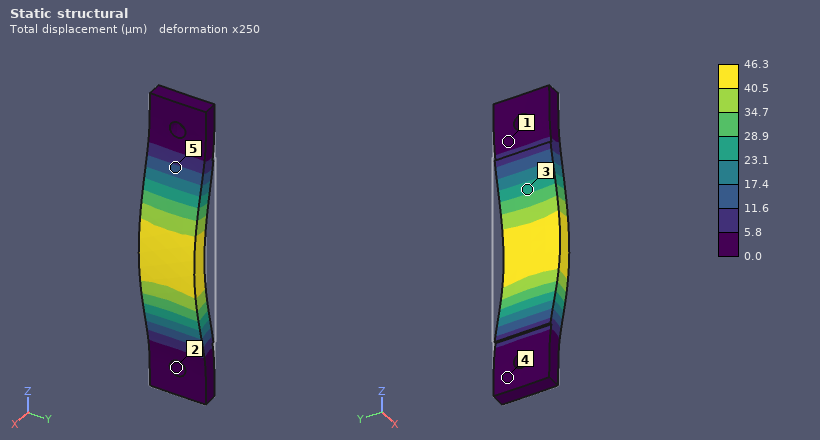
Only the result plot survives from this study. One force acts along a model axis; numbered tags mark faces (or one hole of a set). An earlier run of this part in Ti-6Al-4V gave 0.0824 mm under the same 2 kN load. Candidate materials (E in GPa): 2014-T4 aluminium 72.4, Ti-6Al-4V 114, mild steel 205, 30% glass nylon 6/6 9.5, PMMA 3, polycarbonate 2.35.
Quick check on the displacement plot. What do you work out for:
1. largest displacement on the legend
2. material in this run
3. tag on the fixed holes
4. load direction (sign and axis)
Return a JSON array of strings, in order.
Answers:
["46.3 µm", "mild steel", "2", "+X"]
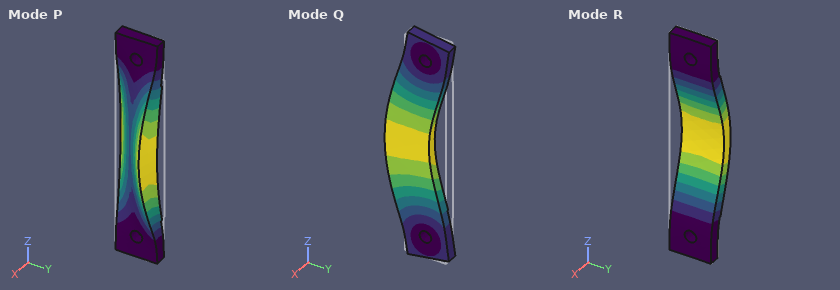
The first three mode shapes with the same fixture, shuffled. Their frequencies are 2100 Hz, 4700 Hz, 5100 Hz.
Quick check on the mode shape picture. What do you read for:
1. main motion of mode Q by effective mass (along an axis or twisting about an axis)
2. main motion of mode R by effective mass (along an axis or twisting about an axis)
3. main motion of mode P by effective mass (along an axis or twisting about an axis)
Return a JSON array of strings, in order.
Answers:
["along Y", "along X", "twisting about Z"]
